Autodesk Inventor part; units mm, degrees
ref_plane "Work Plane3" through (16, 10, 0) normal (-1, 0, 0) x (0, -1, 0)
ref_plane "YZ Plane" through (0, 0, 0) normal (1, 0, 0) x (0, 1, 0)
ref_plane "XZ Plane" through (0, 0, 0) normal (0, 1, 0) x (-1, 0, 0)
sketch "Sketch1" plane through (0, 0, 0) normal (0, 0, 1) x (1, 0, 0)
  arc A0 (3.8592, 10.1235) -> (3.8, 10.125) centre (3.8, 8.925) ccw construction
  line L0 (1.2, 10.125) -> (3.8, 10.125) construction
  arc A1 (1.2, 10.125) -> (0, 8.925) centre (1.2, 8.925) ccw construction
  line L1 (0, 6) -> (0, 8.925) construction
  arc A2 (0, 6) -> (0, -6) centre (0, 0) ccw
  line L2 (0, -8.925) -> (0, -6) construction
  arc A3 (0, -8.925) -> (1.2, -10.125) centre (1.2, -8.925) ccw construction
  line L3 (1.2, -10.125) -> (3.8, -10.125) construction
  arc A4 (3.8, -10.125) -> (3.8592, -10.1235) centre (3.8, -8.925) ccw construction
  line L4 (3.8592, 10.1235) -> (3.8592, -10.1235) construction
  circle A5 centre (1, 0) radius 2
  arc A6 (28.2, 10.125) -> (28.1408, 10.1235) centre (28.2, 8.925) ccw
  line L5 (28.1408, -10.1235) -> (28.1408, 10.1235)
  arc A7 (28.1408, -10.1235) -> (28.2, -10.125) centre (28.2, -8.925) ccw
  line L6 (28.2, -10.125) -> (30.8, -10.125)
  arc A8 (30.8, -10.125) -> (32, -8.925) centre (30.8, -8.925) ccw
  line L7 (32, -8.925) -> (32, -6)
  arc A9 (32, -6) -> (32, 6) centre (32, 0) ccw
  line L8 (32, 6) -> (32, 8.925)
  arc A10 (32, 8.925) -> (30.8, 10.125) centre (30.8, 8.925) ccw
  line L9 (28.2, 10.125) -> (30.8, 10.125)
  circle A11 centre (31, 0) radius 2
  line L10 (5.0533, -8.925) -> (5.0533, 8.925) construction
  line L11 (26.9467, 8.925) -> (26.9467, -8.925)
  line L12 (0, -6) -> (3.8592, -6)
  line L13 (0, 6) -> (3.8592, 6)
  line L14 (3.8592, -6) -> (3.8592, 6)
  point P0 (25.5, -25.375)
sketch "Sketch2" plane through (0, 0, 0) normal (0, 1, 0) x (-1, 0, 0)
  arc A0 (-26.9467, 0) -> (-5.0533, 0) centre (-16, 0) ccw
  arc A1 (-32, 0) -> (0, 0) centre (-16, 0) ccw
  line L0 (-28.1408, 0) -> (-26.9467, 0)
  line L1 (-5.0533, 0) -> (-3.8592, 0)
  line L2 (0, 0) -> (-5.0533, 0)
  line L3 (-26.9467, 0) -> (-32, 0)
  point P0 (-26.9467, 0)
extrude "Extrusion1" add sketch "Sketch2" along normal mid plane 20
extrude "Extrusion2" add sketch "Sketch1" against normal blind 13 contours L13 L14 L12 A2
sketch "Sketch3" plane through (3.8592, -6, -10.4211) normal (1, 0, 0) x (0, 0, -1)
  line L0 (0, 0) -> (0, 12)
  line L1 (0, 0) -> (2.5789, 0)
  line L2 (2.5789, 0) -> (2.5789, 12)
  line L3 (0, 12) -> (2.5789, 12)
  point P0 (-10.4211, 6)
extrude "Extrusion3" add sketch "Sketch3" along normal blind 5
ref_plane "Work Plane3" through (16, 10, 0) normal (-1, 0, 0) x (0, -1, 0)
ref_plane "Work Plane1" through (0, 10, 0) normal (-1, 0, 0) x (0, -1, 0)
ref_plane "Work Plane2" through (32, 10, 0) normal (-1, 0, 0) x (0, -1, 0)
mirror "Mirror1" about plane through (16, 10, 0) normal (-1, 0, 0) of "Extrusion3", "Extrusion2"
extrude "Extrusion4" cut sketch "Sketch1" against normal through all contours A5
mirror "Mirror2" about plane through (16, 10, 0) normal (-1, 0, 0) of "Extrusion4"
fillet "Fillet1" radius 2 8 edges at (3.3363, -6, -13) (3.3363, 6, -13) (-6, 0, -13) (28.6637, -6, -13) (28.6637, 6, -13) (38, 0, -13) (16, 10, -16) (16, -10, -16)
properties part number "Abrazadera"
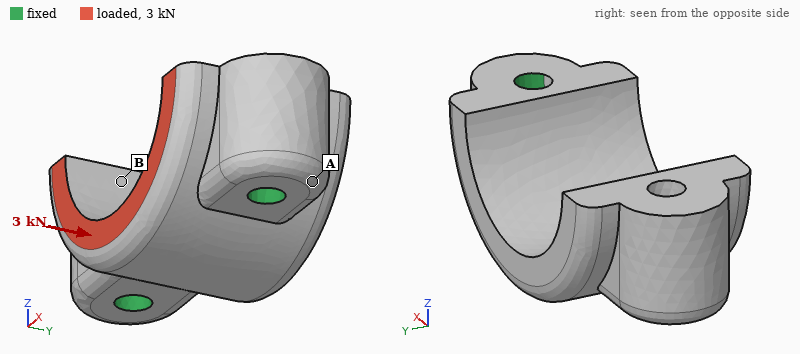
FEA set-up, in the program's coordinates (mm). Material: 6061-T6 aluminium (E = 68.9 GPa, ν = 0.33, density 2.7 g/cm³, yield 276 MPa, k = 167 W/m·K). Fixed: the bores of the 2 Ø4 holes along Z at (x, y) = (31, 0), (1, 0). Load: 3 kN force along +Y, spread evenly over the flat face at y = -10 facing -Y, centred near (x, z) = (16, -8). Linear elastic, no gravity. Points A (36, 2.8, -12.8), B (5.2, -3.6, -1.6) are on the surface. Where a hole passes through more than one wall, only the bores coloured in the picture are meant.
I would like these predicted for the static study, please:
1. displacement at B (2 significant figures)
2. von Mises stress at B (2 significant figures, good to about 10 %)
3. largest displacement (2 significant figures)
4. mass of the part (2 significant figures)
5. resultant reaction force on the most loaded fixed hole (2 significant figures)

5.3 µm
29 MPa
12 µm
16 g
1.5 kN
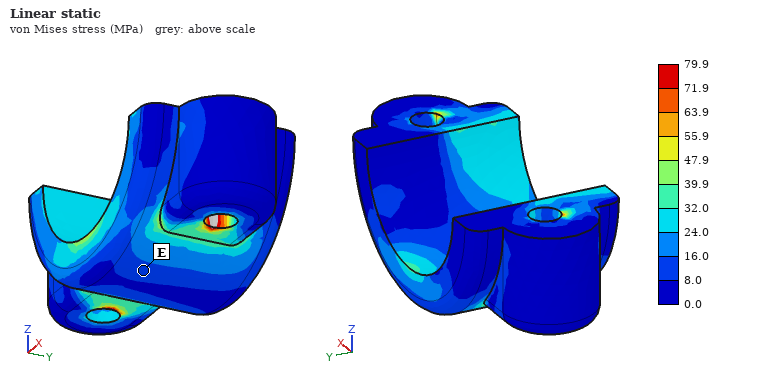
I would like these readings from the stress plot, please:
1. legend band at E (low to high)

8.0 to 16.0 MPa
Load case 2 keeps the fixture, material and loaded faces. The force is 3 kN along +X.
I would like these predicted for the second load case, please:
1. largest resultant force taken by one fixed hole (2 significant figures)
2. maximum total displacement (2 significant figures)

1.7 kN
18 µm
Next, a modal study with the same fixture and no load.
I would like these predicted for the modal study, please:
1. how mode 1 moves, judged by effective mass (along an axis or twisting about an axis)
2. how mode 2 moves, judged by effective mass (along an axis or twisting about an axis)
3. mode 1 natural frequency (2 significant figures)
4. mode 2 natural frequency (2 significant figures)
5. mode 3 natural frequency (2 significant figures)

along Y
along Z
29 kHz
36 kHz
41 kHz
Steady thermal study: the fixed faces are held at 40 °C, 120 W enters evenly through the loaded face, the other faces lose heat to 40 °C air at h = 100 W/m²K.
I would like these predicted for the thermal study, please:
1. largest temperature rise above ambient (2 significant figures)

51 K
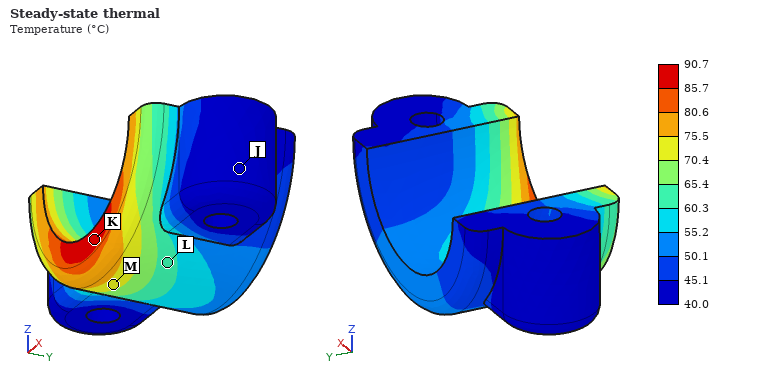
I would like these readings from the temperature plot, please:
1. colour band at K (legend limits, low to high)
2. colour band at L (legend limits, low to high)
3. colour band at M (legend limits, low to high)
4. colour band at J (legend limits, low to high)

85.7 to 90.7 °C
60.3 to 65.4 °C
70.4 to 75.5 °C
40.0 to 45.1 °C
